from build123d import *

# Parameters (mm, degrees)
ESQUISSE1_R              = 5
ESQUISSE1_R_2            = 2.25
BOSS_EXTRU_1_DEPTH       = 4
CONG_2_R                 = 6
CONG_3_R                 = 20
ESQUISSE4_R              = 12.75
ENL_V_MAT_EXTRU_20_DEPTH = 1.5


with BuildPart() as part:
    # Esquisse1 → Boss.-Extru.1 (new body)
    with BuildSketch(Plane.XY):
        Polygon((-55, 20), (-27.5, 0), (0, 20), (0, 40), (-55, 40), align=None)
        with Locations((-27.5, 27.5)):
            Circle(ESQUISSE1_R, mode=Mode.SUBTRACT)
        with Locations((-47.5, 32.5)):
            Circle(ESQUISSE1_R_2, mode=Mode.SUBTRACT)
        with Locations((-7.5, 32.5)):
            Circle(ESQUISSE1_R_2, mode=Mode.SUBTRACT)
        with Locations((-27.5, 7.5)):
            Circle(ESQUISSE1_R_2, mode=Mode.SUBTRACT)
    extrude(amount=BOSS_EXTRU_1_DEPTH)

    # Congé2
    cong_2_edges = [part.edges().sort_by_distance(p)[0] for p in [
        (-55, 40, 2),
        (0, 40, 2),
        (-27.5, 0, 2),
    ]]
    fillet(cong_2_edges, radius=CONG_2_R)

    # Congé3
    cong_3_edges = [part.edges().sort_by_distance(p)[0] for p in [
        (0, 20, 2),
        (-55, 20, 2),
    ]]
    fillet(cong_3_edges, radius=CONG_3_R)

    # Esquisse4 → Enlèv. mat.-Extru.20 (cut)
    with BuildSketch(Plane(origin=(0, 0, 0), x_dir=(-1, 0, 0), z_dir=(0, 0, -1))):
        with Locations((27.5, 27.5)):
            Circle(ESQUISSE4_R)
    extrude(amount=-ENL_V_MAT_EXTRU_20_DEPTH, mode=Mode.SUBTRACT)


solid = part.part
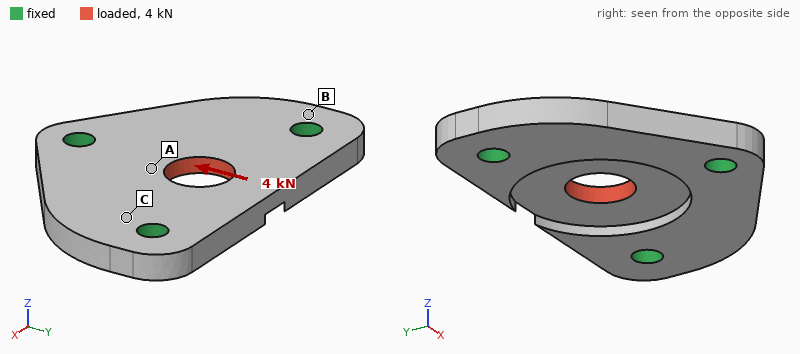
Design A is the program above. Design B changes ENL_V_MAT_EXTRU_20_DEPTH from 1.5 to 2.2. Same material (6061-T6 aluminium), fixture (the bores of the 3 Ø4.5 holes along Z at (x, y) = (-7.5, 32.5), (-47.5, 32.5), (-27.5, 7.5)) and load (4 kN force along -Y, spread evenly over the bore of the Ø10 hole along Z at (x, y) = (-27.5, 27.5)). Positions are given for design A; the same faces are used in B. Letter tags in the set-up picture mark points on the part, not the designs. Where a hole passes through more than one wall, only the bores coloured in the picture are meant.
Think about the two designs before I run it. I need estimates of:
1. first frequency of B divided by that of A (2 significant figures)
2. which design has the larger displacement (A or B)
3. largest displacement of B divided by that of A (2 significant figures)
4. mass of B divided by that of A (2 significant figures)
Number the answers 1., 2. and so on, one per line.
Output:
1. 1.0
2. B
3. 1.3
4. 0.94
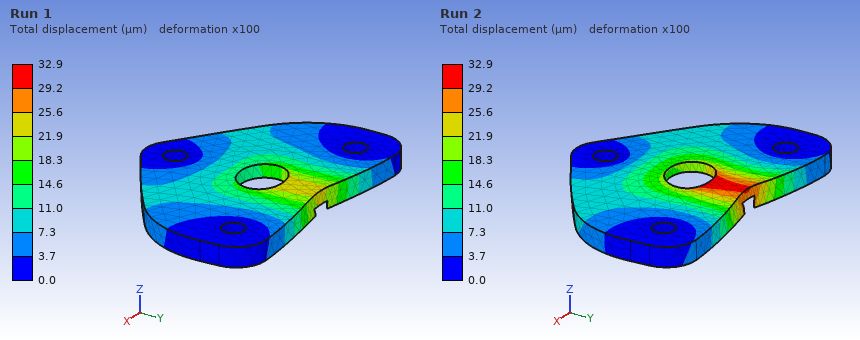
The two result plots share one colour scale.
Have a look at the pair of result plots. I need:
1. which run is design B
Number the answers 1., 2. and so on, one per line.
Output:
1. Run 2
